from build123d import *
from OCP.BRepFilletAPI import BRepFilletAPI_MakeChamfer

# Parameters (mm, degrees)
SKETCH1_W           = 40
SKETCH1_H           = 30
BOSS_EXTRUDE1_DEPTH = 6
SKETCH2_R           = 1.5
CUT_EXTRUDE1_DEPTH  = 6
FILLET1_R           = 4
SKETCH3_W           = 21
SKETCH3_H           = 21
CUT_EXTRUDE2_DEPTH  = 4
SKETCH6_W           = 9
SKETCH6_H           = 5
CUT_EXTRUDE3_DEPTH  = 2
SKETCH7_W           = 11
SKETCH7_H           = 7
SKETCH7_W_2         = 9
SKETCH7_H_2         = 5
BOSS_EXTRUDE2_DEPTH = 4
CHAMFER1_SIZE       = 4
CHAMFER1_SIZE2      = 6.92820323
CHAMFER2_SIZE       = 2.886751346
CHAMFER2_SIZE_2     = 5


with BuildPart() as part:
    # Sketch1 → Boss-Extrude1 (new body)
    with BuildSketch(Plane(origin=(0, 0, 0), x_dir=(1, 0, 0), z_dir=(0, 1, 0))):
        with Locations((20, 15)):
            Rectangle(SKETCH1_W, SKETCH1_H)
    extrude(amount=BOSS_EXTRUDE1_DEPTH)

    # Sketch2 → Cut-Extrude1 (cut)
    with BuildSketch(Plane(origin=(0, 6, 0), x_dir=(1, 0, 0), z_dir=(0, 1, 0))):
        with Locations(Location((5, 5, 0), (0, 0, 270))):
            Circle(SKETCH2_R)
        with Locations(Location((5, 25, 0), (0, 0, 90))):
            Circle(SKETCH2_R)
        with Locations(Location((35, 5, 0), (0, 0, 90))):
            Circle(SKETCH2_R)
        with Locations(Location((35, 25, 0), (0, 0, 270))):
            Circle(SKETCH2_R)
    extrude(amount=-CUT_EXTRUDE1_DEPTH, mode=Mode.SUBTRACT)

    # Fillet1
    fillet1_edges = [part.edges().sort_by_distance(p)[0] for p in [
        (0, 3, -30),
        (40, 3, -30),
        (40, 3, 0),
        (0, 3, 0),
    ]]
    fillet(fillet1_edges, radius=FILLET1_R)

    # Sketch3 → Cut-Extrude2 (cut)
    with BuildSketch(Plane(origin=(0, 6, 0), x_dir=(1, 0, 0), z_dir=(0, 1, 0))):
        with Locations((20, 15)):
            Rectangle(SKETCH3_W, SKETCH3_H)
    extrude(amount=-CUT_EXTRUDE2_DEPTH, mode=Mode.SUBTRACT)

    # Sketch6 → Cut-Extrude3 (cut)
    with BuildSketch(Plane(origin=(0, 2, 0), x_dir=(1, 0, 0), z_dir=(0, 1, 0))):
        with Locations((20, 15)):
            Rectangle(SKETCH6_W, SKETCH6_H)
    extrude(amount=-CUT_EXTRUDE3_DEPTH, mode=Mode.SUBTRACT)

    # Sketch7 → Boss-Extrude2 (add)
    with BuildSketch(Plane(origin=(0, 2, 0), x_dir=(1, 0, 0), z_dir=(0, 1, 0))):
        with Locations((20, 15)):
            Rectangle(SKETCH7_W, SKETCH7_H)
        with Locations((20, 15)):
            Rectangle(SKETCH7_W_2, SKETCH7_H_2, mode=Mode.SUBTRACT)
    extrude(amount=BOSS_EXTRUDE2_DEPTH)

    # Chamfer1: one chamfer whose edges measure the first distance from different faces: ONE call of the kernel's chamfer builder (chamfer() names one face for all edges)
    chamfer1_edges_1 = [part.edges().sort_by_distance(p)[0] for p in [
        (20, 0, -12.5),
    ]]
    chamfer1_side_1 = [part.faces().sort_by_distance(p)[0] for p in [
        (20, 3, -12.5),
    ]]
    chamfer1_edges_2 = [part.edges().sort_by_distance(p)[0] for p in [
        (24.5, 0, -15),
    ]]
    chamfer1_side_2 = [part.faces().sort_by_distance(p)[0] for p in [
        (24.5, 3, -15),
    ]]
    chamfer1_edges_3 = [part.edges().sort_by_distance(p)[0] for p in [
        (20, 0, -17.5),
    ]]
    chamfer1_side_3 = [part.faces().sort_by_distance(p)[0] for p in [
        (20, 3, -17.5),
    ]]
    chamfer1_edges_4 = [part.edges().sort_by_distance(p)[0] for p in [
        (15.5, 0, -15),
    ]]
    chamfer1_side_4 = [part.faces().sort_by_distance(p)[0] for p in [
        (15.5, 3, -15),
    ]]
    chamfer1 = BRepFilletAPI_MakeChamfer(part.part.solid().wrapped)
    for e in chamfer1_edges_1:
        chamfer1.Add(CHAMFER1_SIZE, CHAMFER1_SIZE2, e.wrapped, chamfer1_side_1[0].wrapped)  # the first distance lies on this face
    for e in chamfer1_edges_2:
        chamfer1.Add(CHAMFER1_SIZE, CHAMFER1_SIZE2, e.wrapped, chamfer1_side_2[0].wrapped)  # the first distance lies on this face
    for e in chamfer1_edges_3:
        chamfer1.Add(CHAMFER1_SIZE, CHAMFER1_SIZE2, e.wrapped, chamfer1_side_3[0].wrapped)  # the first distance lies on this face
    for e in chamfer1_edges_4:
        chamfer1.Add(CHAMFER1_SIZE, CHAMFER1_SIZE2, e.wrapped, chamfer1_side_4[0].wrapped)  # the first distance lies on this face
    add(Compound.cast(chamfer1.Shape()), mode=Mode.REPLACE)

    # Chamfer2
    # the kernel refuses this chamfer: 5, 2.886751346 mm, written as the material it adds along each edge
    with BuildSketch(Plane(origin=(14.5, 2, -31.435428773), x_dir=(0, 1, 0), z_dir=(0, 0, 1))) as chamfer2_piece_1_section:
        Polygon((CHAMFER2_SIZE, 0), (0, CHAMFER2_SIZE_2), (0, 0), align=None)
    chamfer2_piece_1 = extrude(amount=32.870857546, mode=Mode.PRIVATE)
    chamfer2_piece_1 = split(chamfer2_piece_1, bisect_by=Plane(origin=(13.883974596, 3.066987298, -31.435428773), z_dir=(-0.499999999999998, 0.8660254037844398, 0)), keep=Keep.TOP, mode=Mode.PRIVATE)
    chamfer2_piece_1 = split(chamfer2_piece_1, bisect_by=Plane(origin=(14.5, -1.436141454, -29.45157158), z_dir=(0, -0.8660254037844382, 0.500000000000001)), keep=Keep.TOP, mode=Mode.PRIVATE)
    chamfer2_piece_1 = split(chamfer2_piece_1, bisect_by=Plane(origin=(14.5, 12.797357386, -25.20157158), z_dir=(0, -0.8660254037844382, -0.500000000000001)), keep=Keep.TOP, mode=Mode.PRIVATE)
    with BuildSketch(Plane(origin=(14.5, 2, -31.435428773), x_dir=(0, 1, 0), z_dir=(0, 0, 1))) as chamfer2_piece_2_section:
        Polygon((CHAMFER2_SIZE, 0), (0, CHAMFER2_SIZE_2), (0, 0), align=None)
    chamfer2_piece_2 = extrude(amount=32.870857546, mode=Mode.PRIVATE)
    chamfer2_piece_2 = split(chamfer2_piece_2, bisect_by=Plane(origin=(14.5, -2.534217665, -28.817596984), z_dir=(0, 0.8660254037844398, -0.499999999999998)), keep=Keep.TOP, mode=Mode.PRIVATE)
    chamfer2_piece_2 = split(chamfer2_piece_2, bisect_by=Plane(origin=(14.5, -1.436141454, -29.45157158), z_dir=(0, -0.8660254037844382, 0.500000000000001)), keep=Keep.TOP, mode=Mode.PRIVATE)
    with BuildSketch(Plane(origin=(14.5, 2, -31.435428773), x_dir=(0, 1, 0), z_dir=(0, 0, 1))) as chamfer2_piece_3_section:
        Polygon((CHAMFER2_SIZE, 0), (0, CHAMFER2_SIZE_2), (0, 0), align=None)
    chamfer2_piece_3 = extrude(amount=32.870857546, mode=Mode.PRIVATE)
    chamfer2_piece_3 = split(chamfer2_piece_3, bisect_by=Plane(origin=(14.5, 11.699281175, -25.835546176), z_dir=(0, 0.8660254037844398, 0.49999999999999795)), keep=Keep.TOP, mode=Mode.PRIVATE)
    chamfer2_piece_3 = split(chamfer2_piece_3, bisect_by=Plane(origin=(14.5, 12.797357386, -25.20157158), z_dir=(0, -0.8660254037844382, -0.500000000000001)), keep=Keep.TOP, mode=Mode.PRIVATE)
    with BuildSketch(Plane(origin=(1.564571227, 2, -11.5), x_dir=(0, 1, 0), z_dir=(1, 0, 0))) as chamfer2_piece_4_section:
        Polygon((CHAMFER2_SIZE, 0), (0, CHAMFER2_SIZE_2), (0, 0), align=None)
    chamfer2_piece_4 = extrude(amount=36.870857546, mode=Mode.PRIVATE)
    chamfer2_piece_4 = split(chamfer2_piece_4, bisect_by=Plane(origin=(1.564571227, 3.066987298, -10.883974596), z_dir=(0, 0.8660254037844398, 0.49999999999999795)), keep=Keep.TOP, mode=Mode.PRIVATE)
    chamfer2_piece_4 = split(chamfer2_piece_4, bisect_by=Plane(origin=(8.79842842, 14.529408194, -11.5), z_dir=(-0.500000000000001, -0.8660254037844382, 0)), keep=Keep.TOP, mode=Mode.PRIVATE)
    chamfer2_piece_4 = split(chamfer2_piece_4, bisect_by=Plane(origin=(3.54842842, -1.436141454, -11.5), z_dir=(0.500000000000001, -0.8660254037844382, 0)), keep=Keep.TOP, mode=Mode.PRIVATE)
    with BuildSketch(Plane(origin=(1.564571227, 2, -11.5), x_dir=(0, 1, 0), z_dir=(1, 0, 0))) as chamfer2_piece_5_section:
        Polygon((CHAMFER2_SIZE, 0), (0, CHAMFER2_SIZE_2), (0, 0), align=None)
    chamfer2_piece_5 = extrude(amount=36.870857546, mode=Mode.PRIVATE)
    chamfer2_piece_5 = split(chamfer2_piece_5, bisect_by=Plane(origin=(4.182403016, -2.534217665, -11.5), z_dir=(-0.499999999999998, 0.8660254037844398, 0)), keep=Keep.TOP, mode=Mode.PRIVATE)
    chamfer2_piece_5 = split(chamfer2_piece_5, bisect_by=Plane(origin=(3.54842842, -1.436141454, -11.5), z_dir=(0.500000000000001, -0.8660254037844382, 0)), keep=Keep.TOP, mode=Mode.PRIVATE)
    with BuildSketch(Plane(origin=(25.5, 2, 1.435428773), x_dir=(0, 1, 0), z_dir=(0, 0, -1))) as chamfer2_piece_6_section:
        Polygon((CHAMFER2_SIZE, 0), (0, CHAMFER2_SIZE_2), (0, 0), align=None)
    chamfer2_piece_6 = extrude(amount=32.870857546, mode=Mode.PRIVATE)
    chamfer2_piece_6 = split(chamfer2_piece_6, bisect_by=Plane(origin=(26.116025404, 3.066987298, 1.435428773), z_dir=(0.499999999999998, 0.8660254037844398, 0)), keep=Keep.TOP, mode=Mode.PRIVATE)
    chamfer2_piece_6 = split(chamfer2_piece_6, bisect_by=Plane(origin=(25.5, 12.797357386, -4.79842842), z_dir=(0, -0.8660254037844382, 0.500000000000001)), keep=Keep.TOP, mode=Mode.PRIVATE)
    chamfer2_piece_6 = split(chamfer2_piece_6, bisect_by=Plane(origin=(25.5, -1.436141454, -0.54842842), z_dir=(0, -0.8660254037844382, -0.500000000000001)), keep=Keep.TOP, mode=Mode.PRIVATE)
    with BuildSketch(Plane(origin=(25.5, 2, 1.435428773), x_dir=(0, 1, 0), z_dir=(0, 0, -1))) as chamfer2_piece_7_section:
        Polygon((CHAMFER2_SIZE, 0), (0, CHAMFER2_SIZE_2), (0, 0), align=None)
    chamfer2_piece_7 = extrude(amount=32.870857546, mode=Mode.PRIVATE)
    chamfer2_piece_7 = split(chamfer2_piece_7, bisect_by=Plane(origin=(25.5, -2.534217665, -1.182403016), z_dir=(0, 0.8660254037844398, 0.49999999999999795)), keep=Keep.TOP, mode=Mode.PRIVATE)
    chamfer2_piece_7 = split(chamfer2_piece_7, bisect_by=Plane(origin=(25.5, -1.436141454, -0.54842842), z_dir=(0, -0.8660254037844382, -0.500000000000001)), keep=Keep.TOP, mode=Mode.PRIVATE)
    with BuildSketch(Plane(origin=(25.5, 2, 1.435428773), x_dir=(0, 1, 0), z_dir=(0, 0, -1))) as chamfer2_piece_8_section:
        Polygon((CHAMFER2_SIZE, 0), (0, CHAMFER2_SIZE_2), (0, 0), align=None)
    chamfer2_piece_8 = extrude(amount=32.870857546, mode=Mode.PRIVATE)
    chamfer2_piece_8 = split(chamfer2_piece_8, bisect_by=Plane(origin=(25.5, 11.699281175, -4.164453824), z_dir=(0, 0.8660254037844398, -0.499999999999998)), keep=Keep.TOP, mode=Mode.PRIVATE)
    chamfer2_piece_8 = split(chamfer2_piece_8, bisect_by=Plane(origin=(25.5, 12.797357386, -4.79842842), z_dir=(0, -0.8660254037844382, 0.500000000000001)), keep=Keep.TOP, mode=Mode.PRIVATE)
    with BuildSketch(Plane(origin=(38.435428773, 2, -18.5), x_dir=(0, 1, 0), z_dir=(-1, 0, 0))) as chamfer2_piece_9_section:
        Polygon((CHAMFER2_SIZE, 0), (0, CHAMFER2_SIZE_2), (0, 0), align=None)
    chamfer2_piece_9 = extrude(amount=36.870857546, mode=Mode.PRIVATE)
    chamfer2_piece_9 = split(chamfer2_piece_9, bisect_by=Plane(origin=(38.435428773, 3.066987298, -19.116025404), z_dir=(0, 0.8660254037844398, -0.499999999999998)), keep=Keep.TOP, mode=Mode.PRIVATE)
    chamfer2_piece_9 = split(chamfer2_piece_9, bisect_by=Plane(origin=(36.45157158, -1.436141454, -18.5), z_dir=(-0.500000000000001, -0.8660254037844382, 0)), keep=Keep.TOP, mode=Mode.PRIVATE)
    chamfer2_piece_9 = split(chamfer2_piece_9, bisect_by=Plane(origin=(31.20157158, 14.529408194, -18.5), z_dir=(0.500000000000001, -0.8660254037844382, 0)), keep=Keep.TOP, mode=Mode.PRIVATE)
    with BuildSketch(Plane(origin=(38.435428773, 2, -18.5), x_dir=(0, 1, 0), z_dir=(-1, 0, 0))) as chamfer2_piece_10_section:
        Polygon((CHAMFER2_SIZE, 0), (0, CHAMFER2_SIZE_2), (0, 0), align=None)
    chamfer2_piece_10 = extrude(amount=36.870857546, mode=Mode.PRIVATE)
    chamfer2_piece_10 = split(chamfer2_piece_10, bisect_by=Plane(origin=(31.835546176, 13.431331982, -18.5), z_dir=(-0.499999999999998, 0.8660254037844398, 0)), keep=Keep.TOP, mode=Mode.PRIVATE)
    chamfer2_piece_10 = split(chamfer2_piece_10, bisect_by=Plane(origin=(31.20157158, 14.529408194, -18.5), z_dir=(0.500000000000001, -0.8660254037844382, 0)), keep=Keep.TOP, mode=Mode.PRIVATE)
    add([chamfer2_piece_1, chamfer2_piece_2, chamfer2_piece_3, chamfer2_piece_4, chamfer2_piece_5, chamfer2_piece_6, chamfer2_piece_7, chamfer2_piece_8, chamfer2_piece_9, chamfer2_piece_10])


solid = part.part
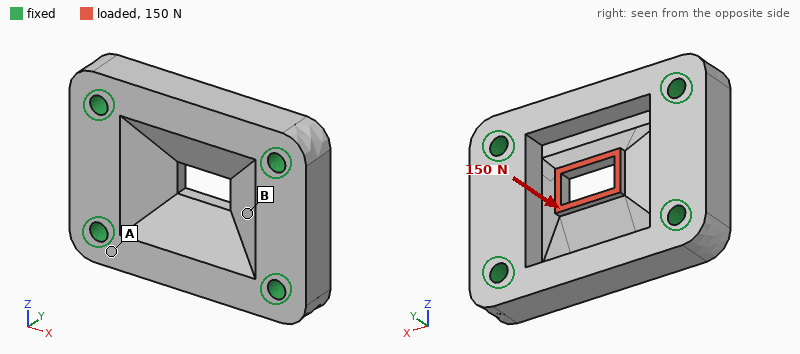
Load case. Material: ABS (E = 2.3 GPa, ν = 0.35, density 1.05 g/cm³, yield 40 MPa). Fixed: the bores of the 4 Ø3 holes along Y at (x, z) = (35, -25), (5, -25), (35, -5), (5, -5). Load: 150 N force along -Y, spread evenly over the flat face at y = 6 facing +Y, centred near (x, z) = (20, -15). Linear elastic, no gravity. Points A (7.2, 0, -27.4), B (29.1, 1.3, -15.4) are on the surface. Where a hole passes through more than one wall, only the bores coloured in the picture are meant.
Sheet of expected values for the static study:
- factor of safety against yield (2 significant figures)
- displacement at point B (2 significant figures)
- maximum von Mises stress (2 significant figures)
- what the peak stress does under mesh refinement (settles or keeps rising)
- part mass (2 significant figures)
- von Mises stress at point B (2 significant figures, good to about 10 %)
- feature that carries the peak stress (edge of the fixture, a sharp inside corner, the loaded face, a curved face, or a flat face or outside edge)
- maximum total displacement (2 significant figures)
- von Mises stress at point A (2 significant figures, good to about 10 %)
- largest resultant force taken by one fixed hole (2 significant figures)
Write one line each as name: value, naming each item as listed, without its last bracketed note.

factor of safety against yield: 1.0
displacement at point B: 0.046 mm
maximum von Mises stress: 40 MPa
what the peak stress does under mesh refinement: settles
part mass: 5.2 g
von Mises stress at point B: 9.4 MPa
feature that carries the peak stress: the loaded face
maximum total displacement: 0.22 mm
von Mises stress at point A: 3.2 MPa
largest resultant force taken by one fixed hole: 54 N
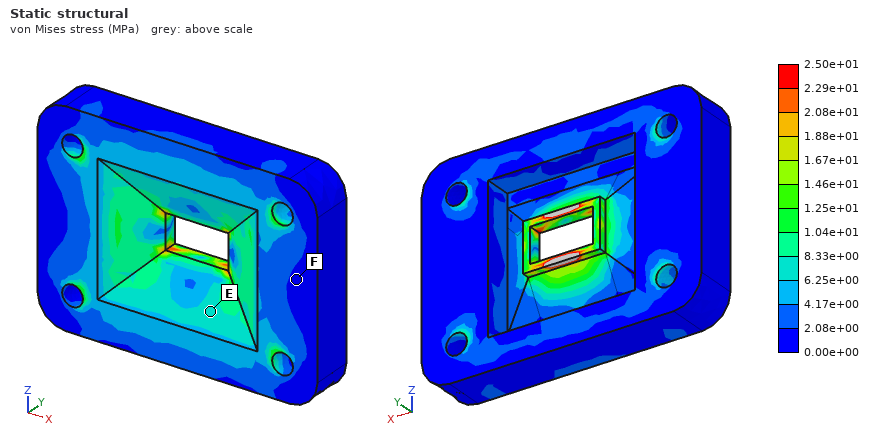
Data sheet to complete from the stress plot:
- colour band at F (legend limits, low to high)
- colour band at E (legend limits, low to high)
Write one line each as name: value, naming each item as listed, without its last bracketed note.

colour band at F: 0.00e+00 to 2.08e+00 MPa
colour band at E: 6.25e+00 to 8.33e+00 MPa
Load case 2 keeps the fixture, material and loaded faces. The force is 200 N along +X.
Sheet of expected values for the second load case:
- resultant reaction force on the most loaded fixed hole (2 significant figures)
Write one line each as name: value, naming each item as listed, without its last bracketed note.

resultant reaction force on the most loaded fixed hole: 57 N
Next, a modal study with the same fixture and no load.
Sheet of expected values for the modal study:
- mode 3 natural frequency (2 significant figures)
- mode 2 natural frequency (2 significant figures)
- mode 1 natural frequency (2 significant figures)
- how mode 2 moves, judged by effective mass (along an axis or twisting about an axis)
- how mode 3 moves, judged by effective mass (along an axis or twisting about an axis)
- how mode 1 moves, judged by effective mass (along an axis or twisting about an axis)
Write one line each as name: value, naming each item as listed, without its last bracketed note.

mode 3 natural frequency: 11 kHz
mode 2 natural frequency: 8700 Hz
mode 1 natural frequency: 8200 Hz
how mode 2 moves, judged by effective mass: twisting about X
how mode 3 moves, judged by effective mass: along Z
how mode 1 moves, judged by effective mass: along Y
